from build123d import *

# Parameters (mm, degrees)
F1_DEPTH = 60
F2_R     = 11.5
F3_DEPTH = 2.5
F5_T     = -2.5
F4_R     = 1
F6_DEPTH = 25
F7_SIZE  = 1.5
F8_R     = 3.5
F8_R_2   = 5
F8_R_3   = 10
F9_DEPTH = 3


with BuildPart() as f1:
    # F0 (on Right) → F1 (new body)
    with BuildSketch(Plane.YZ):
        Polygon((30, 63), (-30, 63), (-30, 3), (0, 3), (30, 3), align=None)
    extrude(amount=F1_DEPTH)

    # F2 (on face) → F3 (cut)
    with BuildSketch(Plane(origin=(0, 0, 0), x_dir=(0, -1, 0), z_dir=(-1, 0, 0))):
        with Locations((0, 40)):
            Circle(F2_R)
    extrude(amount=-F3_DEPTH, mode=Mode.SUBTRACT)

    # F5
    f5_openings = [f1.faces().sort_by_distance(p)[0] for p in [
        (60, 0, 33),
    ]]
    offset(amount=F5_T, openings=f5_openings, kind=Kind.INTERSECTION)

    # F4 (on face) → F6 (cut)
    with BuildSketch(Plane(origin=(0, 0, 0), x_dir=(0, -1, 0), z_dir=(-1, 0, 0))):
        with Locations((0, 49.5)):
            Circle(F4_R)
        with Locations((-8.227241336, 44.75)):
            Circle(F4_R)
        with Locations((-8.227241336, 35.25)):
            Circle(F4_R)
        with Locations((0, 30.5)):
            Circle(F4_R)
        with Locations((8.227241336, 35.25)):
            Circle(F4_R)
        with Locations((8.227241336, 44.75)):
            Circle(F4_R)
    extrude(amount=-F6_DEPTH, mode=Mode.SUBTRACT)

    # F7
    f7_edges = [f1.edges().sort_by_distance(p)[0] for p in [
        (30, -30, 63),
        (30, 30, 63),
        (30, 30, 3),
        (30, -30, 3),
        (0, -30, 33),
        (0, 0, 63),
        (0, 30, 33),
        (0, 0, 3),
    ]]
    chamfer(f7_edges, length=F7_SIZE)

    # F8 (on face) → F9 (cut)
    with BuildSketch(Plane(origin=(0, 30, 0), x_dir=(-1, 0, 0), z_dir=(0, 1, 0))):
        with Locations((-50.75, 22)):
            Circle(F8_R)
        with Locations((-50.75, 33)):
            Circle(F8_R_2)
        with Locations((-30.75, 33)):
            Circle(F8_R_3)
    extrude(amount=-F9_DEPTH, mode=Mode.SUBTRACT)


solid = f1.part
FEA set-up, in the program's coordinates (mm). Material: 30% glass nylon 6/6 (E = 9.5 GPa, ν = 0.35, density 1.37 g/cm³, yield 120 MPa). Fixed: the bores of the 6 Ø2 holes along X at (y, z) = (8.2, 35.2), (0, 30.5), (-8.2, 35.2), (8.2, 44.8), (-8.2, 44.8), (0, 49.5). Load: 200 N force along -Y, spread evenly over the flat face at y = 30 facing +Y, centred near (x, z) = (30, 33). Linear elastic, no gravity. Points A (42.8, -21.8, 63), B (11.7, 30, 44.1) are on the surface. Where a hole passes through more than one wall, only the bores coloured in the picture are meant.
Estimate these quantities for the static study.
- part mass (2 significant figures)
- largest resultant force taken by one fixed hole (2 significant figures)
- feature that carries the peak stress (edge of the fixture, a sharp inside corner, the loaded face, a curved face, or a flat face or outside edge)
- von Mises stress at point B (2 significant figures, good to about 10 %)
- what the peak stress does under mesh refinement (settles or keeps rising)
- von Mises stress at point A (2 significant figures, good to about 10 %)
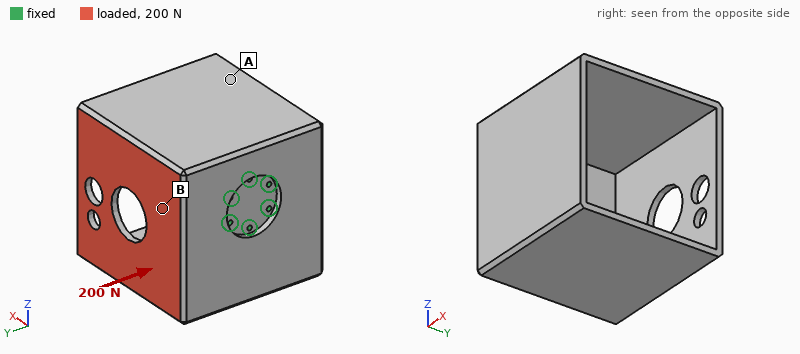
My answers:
56 g
190 N
edge of the fixture
7.4 MPa
keeps rising
3.3 MPa
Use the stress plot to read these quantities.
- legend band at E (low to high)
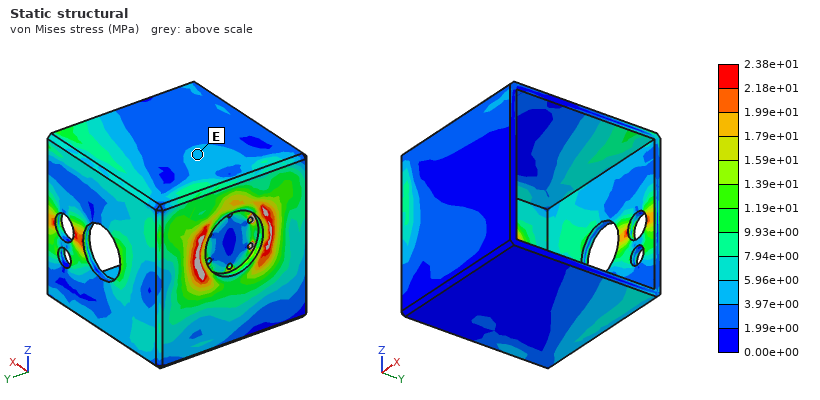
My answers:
3.97e+00 to 5.96e+00 MPa
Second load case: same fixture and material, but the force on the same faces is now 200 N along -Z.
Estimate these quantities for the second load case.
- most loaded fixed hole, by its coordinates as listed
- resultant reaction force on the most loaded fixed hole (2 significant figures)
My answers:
(0, 49.5)
230 N
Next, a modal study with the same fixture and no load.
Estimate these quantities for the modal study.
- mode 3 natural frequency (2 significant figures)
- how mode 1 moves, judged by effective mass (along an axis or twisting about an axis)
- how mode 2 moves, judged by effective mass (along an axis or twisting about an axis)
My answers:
650 Hz
along Z
along Y
